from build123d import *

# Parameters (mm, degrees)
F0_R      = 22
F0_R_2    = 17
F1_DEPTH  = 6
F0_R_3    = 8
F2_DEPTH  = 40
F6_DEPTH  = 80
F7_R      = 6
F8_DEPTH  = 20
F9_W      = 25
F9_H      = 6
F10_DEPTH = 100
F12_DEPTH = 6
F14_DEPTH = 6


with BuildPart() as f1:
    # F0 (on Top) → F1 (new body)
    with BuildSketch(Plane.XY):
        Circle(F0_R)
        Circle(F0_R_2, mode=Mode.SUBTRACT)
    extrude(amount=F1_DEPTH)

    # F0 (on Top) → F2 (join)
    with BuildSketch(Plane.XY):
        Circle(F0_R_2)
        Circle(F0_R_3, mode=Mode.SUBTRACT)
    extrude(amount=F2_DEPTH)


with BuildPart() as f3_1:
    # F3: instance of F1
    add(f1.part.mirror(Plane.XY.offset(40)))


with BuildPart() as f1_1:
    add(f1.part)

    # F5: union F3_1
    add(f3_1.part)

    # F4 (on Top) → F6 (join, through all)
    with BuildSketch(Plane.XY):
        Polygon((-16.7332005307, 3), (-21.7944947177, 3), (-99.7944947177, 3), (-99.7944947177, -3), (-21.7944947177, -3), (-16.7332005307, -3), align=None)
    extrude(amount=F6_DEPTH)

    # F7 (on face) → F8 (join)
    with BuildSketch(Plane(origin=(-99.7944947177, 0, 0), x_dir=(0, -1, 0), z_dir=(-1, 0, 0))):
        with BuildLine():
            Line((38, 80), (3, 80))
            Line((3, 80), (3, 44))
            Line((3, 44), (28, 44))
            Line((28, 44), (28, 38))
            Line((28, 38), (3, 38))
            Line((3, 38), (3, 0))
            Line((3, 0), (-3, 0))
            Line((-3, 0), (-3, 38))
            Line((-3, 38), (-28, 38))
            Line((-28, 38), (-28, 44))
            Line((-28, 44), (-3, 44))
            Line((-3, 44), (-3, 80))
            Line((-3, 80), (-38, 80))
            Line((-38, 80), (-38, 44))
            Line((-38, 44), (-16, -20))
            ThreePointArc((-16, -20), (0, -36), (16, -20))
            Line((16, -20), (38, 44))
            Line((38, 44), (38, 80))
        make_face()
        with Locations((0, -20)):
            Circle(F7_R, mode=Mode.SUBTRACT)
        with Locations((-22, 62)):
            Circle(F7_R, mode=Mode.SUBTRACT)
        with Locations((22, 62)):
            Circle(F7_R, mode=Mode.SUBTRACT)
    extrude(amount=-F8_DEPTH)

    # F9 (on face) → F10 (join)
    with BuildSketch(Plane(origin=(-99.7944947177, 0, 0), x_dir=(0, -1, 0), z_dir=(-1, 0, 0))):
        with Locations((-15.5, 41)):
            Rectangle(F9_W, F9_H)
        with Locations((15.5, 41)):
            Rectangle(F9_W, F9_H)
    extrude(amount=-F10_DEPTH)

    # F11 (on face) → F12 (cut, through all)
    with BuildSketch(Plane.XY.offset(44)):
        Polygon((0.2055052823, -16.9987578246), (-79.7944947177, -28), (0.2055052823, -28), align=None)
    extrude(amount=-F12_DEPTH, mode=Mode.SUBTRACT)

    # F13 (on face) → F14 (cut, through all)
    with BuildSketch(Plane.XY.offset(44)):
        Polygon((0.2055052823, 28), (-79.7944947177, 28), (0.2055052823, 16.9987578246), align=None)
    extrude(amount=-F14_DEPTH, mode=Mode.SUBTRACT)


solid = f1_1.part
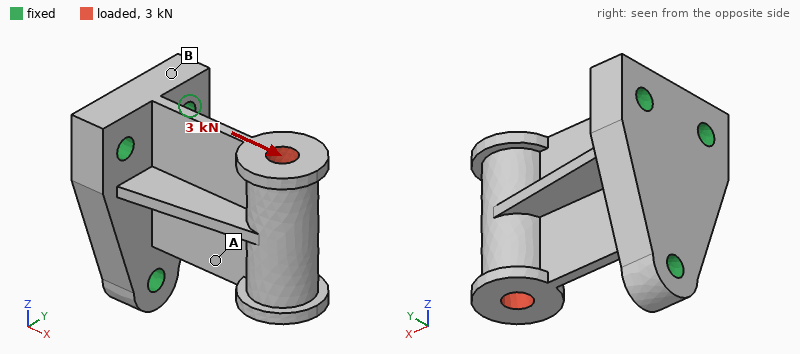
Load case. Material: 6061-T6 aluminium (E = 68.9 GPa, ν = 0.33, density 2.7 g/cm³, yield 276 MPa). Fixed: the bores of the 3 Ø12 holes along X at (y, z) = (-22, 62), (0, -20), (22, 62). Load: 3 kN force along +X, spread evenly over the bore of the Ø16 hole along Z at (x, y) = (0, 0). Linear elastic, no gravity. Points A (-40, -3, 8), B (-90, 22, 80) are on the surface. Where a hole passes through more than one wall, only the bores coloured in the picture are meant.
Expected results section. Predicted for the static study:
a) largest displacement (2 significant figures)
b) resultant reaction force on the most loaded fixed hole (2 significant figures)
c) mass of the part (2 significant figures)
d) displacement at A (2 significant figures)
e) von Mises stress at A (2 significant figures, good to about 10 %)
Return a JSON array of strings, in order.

["8.2 µm", "1.2 kN", "640 g", "5.1 µm", "4.7 MPa"]
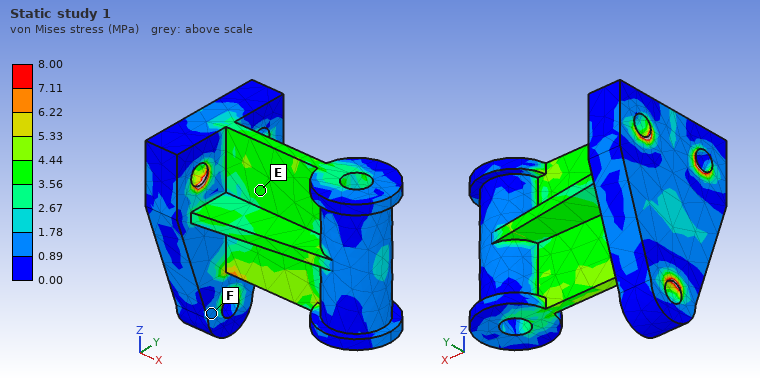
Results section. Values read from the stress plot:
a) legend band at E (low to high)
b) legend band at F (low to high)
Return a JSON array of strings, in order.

["3.56 to 4.44 MPa", "0.89 to 1.78 MPa"]
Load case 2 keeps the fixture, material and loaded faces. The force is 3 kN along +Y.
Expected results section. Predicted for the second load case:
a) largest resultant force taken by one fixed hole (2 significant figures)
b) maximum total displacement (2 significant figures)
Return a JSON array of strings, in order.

["4.9 kN", "0.28 mm"]
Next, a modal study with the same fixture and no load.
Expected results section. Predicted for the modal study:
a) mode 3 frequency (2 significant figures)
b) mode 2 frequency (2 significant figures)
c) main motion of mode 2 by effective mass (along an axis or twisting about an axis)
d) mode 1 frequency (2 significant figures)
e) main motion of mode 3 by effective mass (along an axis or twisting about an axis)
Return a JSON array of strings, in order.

["2300 Hz", "1400 Hz", "along Y", "1100 Hz", "along Z"]
